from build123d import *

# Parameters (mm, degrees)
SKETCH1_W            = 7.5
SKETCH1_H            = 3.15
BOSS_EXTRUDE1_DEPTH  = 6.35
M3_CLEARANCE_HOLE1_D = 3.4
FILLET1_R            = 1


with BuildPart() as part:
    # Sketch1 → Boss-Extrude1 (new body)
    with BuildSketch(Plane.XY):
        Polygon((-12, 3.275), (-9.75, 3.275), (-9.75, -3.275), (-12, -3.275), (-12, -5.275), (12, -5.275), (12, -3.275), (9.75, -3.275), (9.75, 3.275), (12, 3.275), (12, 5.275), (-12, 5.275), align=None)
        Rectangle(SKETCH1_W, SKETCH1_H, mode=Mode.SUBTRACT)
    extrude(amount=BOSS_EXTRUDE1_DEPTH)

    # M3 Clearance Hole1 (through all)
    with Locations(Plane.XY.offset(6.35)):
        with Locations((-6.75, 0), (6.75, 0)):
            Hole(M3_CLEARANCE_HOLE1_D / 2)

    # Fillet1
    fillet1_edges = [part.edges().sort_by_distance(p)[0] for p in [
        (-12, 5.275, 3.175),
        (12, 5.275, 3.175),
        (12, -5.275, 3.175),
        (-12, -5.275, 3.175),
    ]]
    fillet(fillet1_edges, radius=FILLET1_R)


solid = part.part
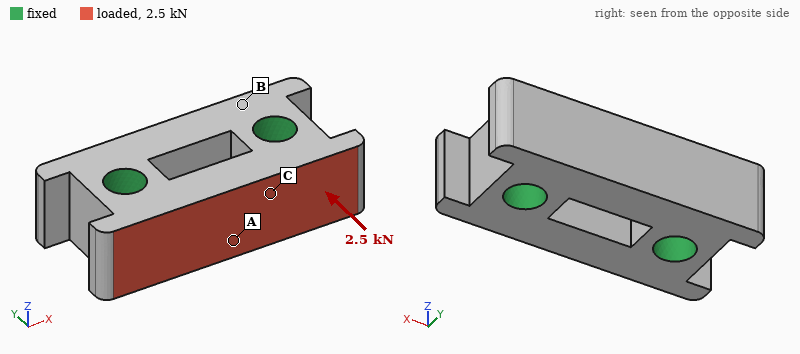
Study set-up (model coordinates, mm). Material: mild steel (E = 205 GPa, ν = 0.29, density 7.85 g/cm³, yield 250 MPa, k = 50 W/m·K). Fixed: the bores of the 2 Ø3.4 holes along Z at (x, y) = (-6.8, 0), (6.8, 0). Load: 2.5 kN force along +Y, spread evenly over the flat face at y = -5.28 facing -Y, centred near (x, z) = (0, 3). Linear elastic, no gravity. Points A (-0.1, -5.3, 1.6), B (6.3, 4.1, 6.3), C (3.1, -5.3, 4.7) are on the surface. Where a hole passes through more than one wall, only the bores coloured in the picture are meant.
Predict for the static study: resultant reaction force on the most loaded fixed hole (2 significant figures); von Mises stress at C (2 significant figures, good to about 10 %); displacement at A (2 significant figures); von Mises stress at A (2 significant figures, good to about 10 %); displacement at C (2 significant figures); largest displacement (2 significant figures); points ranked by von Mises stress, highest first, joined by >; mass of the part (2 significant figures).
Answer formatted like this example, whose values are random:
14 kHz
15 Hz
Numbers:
1.3 kN
17 MPa
1.7 µm
39 MPa
1.2 µm
1.8 µm
A > C > B
9.0 g
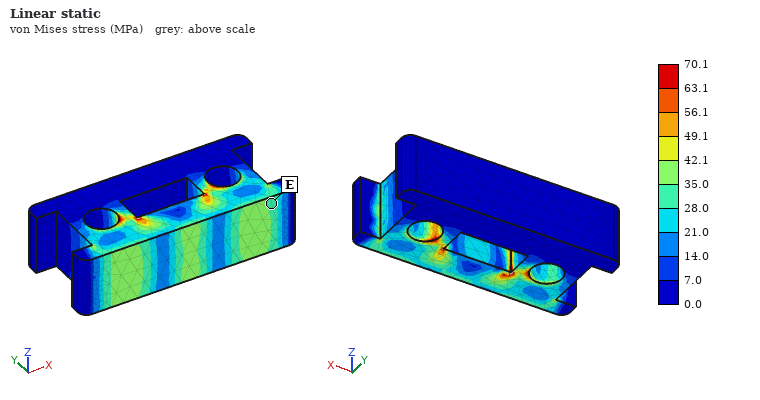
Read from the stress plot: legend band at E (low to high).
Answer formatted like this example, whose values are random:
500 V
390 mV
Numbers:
28.0 to 35.0 MPa
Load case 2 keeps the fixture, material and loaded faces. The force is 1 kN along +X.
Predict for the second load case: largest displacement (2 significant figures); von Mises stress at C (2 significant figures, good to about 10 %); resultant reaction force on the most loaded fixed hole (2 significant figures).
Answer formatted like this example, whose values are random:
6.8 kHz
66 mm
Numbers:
1.7 µm
16 MPa
530 N
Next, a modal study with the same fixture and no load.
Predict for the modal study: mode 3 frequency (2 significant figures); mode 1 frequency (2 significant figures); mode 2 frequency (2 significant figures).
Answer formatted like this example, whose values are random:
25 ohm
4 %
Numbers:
94 kHz
91 kHz
92 kHz
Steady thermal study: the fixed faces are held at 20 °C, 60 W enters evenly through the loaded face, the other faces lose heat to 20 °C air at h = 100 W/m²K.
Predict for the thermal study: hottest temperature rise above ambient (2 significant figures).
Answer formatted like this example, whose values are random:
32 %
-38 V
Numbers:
69 K
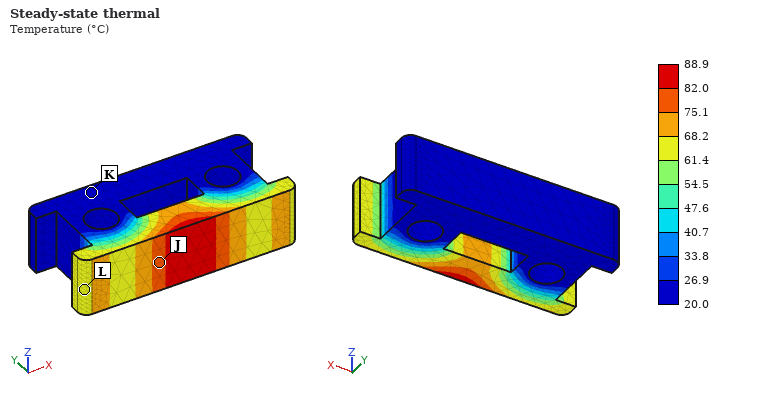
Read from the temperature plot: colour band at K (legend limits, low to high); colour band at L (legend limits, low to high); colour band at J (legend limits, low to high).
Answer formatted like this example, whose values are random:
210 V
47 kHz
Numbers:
20.0 to 26.9 °C
61.4 to 68.2 °C
75.1 to 82.0 °C
